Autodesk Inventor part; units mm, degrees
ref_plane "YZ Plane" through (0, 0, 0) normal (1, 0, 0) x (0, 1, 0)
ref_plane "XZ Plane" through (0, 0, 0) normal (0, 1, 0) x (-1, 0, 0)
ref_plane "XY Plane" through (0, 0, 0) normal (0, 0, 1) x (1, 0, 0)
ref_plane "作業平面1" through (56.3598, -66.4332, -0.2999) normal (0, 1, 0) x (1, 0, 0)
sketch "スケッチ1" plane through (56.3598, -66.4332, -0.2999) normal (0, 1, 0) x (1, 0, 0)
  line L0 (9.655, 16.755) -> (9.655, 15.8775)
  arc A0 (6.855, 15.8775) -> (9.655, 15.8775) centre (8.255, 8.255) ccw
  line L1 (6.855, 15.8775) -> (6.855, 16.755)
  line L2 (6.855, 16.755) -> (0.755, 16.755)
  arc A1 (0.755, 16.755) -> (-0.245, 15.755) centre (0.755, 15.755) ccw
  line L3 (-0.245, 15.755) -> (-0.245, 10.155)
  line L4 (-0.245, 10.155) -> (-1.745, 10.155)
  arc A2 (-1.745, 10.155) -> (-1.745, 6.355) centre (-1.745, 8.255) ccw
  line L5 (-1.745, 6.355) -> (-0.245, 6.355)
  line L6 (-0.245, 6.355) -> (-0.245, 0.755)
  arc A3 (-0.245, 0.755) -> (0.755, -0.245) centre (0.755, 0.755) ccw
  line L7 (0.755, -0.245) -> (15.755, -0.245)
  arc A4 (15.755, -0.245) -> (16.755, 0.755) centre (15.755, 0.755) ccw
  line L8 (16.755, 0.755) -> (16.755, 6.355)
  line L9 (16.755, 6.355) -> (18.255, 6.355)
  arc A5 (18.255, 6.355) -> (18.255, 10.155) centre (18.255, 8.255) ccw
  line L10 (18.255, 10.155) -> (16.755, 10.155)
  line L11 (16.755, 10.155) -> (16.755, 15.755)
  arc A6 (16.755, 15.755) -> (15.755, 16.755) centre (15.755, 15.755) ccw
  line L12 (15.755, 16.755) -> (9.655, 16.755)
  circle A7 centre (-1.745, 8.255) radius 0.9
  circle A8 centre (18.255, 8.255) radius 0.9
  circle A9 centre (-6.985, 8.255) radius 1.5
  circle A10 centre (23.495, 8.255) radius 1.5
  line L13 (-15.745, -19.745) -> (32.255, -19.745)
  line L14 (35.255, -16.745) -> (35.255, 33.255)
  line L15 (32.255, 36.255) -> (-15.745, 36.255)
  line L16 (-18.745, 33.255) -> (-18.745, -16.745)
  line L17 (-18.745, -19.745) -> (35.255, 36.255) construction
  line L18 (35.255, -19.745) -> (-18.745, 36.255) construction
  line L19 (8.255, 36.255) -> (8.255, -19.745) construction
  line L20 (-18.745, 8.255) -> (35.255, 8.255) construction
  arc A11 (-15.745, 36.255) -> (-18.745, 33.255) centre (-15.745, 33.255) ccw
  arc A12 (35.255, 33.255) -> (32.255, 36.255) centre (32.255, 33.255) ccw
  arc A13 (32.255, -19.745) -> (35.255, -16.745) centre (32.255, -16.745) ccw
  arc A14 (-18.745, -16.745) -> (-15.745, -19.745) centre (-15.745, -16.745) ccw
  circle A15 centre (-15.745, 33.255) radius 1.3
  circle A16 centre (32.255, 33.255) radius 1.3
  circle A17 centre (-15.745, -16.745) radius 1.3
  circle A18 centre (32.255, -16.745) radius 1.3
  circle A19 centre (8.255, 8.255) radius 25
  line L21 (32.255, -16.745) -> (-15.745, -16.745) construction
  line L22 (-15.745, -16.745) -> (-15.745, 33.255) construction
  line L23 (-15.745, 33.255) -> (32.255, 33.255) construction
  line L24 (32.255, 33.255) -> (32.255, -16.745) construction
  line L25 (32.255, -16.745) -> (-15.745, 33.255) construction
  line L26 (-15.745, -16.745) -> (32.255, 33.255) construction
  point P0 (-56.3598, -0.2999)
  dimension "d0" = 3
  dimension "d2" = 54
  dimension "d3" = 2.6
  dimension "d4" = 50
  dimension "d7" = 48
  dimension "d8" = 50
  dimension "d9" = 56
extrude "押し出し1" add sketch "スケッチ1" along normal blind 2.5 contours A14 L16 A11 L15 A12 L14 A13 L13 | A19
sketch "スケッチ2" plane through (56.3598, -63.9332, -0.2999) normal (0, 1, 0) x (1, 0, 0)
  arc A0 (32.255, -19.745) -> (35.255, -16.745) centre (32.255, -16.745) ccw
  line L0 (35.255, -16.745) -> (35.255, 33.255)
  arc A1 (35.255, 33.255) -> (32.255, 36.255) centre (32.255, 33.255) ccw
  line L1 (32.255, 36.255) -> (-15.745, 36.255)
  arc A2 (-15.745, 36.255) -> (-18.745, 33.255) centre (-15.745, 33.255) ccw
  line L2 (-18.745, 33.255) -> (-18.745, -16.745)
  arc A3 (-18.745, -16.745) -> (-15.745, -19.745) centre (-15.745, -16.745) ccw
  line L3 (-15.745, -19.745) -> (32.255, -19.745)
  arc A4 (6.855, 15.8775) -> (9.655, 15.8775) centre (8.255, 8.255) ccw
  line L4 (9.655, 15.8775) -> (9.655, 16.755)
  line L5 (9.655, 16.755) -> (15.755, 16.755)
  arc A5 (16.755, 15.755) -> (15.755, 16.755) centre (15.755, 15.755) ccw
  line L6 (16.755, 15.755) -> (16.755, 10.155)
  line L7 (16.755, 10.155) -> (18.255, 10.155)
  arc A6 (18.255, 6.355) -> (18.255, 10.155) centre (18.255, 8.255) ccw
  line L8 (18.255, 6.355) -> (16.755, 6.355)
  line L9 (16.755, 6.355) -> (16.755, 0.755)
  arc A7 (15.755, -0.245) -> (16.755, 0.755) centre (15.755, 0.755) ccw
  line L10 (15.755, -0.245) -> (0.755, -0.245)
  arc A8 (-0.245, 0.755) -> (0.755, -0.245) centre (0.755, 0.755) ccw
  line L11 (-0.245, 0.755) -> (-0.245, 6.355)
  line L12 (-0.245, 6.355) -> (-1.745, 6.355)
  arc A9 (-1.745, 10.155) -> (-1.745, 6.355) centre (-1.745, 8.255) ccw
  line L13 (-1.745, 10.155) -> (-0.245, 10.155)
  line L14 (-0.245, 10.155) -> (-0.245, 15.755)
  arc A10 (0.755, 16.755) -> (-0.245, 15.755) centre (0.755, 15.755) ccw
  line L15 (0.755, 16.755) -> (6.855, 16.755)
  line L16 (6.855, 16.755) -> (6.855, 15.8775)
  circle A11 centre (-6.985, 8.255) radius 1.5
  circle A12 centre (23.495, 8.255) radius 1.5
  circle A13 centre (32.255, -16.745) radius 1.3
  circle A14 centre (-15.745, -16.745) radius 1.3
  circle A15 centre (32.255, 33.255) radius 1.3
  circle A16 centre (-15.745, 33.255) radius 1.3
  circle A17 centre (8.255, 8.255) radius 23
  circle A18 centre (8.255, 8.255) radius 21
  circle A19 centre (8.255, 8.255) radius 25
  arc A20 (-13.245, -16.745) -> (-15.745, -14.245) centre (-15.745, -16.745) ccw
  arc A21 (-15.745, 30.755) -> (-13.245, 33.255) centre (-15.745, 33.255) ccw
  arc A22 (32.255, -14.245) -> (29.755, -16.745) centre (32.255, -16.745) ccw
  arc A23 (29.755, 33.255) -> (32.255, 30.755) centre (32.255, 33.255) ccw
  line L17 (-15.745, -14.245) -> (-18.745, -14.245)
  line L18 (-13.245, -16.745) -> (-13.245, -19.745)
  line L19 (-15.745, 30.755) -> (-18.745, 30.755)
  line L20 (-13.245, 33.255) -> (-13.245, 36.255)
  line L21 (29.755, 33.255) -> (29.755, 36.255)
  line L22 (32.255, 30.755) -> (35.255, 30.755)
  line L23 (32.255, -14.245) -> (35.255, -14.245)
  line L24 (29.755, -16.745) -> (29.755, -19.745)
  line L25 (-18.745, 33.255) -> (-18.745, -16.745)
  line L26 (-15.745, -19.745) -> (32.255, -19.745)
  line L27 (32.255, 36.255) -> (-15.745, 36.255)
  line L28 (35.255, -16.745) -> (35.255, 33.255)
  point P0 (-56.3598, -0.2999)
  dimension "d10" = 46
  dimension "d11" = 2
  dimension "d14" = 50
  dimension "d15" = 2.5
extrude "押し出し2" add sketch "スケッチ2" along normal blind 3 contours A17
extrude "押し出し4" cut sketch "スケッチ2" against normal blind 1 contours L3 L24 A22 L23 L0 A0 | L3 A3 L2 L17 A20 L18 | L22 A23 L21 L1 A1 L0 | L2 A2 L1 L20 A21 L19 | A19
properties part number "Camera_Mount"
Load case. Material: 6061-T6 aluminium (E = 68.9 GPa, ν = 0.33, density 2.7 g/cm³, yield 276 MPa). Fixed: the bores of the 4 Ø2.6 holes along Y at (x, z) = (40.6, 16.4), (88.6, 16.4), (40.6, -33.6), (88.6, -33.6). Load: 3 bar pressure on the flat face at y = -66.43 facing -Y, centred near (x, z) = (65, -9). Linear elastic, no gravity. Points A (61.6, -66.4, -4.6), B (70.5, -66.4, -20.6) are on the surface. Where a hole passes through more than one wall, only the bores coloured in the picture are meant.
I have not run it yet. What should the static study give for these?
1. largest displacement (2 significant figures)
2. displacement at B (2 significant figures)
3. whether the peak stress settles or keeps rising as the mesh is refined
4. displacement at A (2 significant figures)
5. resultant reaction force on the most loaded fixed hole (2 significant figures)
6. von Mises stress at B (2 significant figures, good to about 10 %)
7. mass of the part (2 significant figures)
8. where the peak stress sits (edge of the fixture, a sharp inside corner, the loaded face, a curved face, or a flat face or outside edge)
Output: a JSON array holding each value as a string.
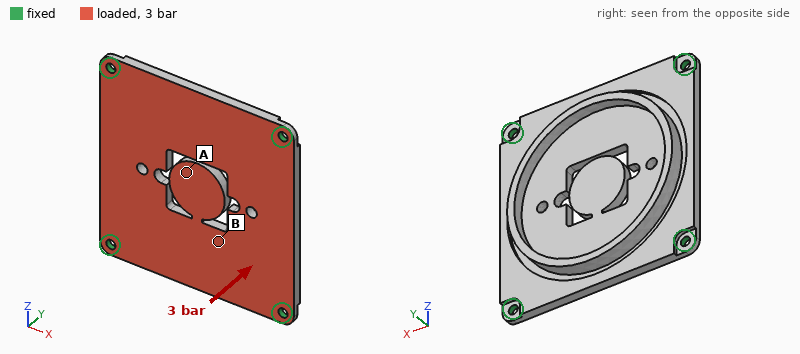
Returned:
["0.46 mm", "0.15 mm", "keeps rising", "0.40 mm", "360 N", "53 MPa", "21 g", "edge of the fixture"]
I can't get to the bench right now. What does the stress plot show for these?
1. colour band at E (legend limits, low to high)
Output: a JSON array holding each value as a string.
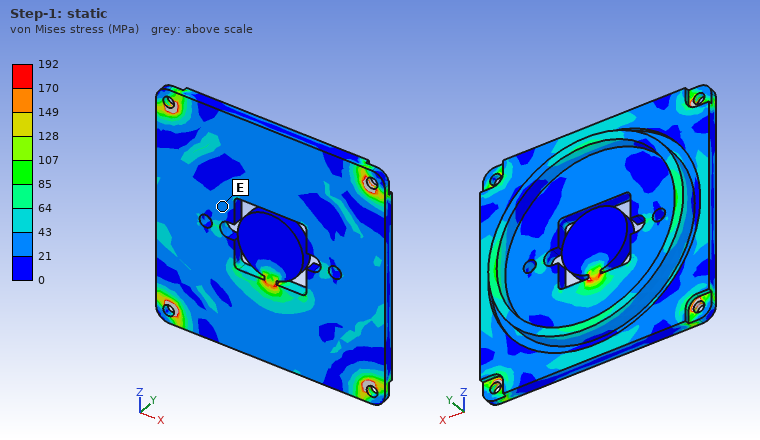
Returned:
["21 to 43 MPa"]
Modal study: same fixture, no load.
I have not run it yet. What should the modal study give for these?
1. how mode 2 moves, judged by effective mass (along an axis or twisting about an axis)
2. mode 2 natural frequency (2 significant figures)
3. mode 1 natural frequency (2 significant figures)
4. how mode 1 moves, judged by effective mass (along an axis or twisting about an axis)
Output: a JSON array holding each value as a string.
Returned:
["along Y", "3800 Hz", "2300 Hz", "along Y"]
